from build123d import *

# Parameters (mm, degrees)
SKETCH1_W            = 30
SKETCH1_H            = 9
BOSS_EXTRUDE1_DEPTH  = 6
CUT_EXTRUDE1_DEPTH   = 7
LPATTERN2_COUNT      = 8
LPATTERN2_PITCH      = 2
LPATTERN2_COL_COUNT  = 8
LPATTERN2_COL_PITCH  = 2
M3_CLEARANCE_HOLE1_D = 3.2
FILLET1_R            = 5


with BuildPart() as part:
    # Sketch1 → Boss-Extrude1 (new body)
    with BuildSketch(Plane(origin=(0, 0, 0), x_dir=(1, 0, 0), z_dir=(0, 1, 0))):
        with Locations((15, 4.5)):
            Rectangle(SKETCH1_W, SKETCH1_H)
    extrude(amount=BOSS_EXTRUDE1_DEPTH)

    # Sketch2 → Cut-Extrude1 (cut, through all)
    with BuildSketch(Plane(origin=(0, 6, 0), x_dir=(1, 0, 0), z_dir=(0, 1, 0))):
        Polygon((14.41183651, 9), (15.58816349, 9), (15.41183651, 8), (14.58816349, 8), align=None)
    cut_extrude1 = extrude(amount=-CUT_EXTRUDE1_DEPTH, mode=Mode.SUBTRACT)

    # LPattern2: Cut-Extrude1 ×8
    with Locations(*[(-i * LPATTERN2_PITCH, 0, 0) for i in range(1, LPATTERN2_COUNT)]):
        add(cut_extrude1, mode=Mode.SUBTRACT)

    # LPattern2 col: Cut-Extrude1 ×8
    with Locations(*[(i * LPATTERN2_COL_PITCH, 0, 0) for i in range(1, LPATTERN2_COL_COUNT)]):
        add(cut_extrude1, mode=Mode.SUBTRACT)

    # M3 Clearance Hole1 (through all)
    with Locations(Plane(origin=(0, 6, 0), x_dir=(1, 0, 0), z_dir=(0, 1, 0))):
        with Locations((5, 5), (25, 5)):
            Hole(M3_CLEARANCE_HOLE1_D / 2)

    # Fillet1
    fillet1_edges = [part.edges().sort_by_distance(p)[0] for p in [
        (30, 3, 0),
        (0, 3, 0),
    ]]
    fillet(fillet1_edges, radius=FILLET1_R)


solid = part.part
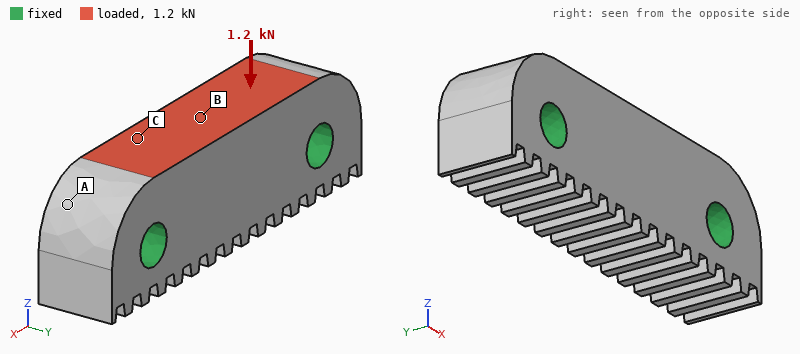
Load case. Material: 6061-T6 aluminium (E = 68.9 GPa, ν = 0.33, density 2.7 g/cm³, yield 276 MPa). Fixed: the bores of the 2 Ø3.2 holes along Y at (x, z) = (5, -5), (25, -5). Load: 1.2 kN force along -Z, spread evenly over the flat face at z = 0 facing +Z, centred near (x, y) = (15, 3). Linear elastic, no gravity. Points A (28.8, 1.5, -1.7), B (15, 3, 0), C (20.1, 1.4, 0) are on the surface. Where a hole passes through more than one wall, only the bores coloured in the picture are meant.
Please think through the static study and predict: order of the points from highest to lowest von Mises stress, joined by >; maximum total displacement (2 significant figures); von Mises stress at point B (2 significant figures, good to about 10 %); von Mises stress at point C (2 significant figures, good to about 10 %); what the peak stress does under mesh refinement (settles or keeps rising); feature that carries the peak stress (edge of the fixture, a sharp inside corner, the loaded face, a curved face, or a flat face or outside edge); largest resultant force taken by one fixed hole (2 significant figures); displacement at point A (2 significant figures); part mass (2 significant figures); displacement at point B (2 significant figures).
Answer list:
B > C > A
4.5 µm
23 MPa
12 MPa
keeps rising
edge of the fixture
620 N
0.68 µm
3.7 g
4.3 µm
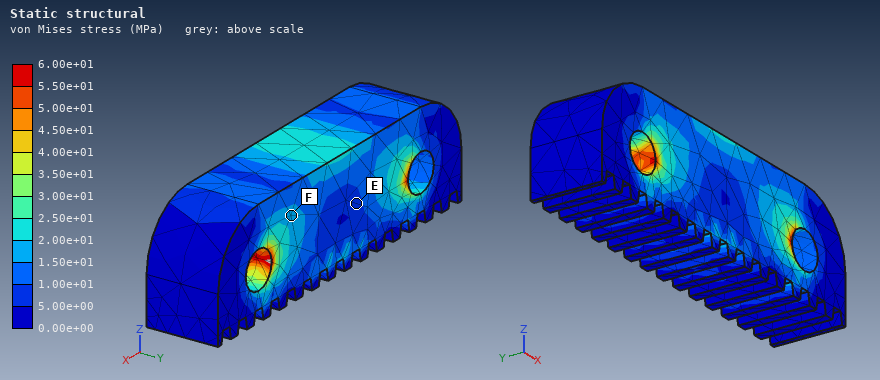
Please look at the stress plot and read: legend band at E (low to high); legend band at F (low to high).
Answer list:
5.00e+00 to 1.00e+01 MPa
1.50e+01 to 2.00e+01 MPa
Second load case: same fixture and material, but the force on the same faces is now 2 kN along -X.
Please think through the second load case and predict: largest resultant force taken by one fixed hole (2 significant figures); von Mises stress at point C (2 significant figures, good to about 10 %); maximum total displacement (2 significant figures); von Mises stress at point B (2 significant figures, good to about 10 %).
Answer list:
1.1 kN
30 MPa
3.5 µm
29 MPa
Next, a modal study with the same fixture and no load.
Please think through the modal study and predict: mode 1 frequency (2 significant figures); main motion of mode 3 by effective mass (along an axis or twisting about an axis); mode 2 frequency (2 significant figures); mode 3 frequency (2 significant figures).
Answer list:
56 kHz
twisting about X
56 kHz
69 kHz
